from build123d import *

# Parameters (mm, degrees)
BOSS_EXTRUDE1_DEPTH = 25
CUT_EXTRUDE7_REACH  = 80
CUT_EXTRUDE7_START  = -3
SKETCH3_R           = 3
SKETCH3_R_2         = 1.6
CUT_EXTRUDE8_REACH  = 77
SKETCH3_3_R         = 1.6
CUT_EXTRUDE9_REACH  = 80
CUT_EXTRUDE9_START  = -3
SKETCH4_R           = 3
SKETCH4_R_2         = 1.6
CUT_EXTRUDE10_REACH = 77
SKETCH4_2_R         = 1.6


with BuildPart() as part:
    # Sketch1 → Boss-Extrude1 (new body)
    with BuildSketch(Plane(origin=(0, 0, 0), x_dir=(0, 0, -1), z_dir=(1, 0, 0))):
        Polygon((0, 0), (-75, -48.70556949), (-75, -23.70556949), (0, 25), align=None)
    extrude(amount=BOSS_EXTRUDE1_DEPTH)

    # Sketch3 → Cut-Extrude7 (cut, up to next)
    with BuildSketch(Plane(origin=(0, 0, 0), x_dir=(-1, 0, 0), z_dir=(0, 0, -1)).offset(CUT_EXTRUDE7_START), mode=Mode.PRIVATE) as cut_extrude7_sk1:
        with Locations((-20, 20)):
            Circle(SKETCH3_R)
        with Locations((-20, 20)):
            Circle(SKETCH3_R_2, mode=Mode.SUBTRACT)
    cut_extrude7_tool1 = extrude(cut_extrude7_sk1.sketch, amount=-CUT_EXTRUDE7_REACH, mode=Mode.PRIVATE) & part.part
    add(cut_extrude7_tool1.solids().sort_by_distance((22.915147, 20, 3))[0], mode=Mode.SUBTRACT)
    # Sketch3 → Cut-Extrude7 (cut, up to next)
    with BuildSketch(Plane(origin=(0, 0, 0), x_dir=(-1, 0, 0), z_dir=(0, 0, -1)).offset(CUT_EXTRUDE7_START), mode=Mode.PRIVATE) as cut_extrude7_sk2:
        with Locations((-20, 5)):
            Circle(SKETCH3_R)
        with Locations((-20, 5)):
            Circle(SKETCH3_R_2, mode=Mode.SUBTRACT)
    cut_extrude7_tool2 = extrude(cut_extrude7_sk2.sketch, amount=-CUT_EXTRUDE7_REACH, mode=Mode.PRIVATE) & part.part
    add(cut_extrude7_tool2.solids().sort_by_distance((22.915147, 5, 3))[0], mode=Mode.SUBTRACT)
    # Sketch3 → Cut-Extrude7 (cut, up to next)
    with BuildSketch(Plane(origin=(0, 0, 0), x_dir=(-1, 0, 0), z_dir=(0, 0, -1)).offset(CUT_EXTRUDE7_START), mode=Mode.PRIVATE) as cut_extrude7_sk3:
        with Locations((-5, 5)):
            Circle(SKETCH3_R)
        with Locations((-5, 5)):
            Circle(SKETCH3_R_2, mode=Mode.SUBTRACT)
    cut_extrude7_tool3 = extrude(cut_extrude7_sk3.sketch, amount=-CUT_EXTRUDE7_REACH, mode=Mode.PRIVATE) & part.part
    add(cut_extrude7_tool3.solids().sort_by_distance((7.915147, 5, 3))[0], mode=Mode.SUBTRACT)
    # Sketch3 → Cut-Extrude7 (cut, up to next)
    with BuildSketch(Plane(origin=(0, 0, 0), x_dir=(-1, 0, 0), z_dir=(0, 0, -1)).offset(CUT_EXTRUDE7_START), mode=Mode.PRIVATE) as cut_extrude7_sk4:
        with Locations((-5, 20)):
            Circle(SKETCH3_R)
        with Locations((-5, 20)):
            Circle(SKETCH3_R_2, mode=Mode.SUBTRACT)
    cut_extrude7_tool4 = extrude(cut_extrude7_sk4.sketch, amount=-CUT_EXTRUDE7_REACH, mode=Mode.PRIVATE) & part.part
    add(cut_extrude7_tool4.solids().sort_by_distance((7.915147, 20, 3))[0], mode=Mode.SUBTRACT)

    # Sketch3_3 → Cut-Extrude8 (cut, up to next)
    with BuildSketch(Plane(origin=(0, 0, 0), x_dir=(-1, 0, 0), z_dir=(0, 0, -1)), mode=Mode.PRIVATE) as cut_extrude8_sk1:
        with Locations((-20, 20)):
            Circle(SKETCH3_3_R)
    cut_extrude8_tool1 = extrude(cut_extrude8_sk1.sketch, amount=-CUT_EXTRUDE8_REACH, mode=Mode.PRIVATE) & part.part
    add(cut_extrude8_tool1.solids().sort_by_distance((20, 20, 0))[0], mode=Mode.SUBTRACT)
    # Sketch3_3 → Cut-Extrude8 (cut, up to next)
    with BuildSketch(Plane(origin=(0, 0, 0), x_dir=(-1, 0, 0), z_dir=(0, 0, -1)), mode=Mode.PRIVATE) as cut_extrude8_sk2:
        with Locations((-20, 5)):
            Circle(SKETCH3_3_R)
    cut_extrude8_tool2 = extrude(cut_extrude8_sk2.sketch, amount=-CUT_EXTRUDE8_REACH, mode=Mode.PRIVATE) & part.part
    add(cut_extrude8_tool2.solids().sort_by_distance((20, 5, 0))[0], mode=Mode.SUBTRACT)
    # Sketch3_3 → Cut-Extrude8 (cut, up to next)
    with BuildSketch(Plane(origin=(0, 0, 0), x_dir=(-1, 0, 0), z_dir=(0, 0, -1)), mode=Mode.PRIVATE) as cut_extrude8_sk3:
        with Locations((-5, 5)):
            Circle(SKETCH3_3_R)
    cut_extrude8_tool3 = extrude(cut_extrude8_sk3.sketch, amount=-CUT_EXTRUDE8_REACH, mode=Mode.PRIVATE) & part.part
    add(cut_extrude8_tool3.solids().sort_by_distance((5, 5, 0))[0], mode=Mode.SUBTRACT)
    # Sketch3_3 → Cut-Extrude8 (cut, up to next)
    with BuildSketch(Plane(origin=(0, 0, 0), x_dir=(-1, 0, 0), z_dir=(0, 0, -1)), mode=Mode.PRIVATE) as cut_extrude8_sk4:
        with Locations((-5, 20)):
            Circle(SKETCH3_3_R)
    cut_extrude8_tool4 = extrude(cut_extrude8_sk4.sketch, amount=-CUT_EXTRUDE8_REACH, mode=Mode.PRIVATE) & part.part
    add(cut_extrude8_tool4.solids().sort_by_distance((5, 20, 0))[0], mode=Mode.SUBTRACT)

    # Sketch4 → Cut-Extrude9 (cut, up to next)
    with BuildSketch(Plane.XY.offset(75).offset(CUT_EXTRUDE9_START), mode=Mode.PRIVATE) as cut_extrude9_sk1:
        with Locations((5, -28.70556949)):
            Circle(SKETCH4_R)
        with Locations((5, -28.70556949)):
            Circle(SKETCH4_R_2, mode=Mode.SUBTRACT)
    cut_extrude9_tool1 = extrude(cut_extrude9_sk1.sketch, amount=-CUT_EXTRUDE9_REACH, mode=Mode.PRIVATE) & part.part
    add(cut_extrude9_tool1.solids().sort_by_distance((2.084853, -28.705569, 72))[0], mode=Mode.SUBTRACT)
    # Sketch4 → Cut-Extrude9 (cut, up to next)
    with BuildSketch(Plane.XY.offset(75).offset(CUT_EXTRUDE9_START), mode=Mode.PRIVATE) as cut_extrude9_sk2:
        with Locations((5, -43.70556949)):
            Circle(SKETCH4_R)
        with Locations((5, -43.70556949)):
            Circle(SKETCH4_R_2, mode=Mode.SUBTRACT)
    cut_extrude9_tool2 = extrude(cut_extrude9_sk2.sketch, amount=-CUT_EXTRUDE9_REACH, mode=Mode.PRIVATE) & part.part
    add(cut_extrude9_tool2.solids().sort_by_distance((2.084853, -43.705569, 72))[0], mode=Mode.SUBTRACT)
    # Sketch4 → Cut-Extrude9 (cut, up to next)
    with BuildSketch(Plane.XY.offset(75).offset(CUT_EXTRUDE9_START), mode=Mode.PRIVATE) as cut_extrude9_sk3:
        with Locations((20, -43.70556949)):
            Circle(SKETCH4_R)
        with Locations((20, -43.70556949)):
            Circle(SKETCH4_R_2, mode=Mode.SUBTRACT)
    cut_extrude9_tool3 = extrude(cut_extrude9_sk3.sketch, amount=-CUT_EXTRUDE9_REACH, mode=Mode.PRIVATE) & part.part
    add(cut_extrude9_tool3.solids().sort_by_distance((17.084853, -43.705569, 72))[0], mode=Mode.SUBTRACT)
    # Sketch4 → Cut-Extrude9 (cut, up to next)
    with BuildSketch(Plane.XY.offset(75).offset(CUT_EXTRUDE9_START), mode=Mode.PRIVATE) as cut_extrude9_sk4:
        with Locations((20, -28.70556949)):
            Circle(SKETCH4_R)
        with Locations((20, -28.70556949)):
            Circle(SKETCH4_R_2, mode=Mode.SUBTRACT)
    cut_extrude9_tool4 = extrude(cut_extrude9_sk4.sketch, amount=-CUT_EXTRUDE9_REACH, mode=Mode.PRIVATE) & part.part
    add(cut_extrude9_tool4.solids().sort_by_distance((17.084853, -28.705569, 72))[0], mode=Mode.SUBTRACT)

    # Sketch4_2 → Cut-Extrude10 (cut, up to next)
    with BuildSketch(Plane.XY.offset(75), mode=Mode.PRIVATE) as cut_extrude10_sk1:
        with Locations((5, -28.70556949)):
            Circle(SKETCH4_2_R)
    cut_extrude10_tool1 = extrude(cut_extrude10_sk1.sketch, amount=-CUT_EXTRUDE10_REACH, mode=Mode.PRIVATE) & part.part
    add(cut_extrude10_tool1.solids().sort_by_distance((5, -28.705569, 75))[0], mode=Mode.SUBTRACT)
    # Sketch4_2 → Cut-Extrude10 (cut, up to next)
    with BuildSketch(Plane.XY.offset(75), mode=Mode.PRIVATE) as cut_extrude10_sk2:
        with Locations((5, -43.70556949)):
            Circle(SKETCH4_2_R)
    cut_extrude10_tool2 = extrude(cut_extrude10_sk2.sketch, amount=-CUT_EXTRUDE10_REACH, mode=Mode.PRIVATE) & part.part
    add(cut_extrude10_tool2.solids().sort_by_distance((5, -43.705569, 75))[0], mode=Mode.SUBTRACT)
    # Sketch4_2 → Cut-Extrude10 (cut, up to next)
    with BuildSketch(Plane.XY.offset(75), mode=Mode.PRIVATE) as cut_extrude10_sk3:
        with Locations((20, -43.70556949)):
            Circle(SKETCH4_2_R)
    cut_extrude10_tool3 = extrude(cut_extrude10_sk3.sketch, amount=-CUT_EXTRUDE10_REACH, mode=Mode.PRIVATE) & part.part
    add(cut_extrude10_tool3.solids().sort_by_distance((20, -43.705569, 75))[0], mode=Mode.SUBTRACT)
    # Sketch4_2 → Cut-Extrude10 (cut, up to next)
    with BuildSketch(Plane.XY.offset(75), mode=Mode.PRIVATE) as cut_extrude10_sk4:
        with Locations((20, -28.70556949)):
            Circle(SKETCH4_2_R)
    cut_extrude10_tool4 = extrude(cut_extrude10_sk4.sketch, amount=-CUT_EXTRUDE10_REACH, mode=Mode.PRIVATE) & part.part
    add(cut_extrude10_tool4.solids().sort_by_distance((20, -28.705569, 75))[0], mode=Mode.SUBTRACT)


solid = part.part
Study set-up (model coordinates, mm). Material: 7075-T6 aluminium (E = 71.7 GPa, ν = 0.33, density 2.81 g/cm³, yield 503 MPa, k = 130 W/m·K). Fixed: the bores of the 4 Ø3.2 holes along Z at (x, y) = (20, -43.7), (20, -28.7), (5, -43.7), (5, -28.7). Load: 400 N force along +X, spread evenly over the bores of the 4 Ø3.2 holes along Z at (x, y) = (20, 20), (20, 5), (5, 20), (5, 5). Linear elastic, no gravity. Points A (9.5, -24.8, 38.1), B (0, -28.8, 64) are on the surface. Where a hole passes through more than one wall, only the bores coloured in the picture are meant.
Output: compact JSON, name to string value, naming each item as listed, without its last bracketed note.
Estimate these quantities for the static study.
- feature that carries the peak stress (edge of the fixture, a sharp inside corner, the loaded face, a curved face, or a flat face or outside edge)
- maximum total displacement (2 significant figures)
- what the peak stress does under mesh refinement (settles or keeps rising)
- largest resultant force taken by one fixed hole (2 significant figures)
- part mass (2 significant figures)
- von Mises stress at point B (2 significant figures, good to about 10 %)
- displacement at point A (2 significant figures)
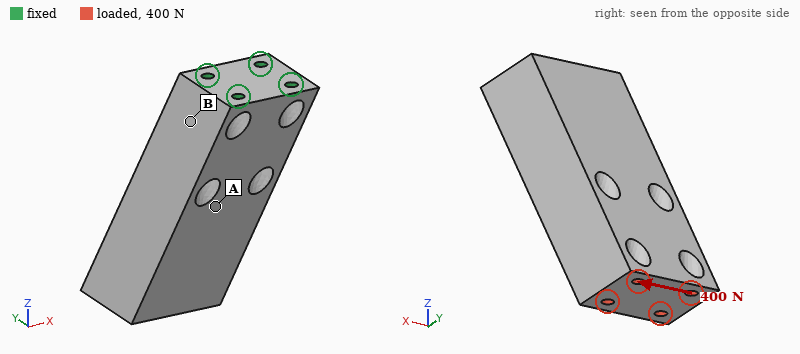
{"feature that carries the peak stress": "edge of the fixture", "maximum total displacement": "92 µm", "what the peak stress does under mesh refinement": "keeps rising", "largest resultant force taken by one fixed hole": "1.3 kN", "part mass": "120 g", "von Mises stress at point B": "21 MPa", "displacement at point A": "25 µm"}
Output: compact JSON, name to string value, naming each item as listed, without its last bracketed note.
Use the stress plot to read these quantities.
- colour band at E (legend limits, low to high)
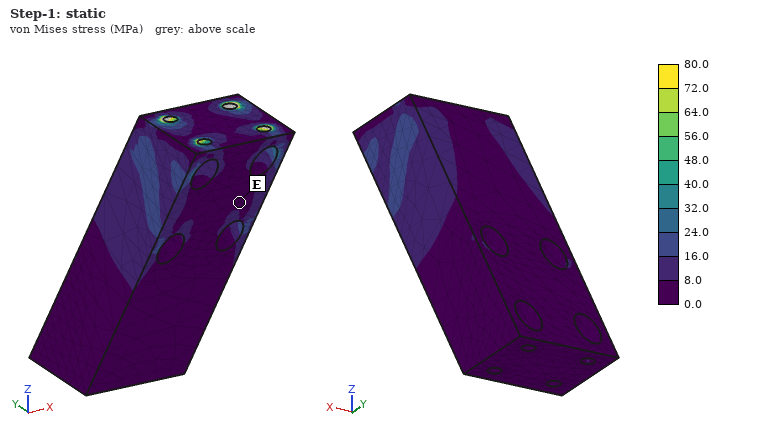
{"colour band at E": "0.0 to 8.0 MPa"}
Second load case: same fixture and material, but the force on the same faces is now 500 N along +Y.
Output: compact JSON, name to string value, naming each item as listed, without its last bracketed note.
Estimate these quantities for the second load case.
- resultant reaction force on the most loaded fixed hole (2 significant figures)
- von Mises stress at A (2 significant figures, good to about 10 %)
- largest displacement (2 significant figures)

{"resultant reaction force on the most loaded fixed hole": "1.2 kN", "von Mises stress at A": "13 MPa", "largest displacement": "0.14 mm"}
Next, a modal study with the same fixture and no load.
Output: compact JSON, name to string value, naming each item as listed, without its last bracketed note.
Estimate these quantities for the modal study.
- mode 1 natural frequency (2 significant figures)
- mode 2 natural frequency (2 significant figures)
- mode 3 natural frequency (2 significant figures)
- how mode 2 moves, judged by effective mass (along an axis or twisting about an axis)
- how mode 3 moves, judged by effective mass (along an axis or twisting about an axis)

{"mode 1 natural frequency": "1600 Hz", "mode 2 natural frequency": "1900 Hz", "mode 3 natural frequency": "7200 Hz", "how mode 2 moves, judged by effective mass": "along X", "how mode 3 moves, judged by effective mass": "twisting about Z"}
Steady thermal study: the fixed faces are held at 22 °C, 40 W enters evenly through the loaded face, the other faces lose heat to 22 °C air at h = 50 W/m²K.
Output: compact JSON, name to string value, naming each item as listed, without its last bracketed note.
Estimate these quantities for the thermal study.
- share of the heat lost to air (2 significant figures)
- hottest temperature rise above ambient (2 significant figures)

{"share of the heat lost to air": "33 %", "hottest temperature rise above ambient": "55 K"}
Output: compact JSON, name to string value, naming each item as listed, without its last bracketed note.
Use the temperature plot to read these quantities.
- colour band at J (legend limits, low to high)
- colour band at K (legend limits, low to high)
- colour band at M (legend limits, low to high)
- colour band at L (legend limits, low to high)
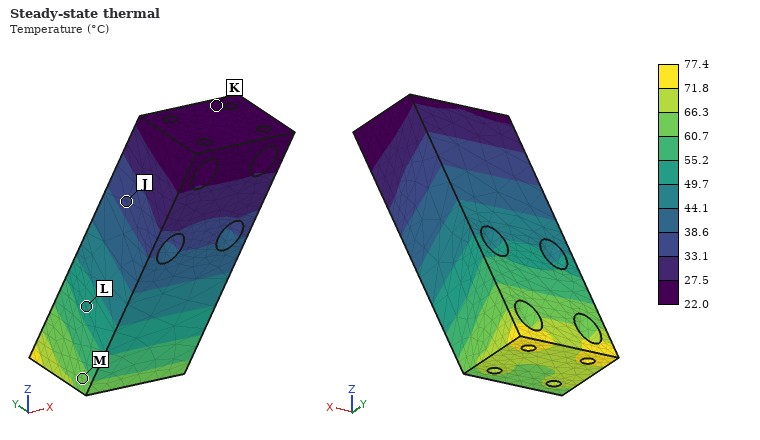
{"colour band at J": "33.1 to 38.6 °C", "colour band at K": "22.0 to 27.5 °C", "colour band at M": "60.7 to 66.3 °C", "colour band at L": "49.7 to 55.2 °C"}
